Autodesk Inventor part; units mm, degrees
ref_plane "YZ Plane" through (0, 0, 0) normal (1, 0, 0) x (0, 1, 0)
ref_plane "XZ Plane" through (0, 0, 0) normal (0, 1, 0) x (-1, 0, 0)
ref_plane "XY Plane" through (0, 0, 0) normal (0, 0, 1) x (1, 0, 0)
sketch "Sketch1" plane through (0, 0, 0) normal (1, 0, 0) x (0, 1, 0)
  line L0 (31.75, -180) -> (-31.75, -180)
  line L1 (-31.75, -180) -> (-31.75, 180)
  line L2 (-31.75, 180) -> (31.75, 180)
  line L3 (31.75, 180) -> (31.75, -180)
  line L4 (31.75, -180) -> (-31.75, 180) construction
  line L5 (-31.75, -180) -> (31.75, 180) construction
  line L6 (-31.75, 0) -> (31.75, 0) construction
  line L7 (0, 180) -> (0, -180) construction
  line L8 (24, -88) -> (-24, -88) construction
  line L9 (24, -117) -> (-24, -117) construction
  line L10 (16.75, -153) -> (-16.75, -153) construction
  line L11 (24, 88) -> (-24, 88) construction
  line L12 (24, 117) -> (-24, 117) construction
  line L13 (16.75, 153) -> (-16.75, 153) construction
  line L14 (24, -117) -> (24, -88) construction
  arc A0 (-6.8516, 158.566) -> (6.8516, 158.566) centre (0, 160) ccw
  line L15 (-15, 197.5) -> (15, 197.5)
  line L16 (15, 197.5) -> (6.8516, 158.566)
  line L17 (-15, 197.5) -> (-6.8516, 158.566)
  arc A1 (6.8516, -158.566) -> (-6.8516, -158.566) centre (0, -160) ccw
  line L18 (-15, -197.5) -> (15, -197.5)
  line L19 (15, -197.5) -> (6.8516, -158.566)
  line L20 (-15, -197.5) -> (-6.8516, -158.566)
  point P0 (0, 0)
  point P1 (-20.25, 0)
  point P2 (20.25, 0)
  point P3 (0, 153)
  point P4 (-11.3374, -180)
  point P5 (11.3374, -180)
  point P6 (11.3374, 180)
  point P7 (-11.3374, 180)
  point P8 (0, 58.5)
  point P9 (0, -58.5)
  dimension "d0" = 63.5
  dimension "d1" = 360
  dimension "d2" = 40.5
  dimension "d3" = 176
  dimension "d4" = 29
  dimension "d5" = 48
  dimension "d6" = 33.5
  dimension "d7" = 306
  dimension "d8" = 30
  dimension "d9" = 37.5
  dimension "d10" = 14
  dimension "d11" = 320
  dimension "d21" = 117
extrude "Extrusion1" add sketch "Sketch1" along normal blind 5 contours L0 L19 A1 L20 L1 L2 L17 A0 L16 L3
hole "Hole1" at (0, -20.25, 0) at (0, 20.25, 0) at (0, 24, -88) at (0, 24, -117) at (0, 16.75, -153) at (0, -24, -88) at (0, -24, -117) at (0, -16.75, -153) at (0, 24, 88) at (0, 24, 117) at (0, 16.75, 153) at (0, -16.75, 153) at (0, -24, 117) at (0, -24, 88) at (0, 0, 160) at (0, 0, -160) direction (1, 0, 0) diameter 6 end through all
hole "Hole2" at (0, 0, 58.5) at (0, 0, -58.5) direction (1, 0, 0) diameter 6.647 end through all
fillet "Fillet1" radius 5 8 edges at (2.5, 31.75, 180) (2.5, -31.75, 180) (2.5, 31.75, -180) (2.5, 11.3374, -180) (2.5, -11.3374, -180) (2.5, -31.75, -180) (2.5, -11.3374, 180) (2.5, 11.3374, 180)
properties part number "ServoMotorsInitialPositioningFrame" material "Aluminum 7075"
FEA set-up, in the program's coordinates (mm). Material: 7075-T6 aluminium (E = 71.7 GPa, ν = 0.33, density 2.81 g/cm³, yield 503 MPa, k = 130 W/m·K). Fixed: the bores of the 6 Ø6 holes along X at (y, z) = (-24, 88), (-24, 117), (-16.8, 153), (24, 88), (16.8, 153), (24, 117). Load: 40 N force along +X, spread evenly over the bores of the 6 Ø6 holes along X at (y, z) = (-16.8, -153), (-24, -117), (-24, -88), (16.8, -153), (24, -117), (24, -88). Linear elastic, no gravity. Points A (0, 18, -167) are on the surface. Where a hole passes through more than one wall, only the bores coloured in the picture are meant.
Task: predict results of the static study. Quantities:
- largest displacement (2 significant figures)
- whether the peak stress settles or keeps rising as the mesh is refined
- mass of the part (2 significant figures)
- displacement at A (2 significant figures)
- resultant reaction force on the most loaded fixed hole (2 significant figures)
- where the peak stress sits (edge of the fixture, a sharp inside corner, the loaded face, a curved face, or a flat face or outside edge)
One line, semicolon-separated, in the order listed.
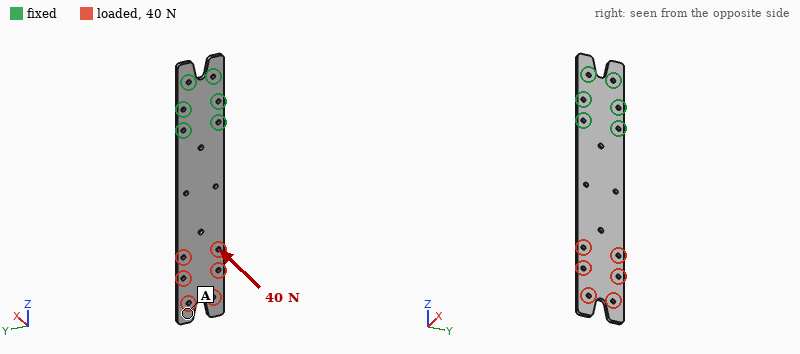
3.7 mm; keeps rising; 300 g; 3.5 mm; 66 N; edge of the fixture
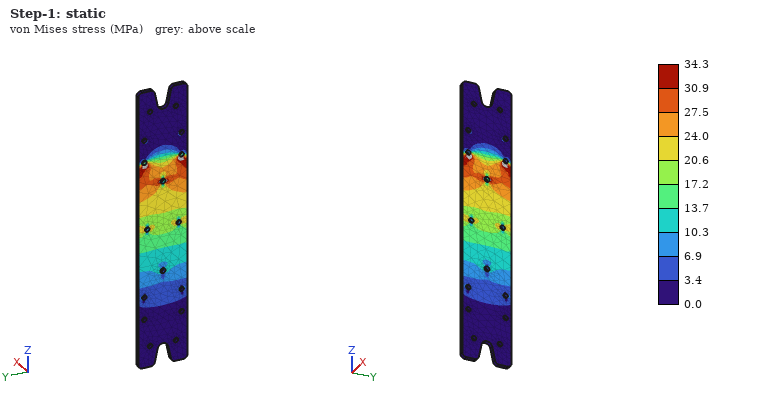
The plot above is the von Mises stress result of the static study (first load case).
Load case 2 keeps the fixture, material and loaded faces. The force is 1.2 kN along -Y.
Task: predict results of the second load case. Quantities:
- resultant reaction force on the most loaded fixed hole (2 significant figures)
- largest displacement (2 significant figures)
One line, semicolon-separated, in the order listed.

4.7 kN; 0.74 mm
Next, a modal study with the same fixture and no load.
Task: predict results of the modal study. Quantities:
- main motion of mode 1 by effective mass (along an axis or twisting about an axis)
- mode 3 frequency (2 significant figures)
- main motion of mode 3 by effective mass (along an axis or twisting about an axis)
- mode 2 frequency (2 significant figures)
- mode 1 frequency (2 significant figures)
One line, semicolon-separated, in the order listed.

along X; 470 Hz; twisting about Z; 370 Hz; 60 Hz
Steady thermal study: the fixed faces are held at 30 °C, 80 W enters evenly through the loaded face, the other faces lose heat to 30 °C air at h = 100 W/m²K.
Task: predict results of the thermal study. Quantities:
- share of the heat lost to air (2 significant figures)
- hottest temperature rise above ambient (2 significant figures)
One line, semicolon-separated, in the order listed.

97 %; 50 K
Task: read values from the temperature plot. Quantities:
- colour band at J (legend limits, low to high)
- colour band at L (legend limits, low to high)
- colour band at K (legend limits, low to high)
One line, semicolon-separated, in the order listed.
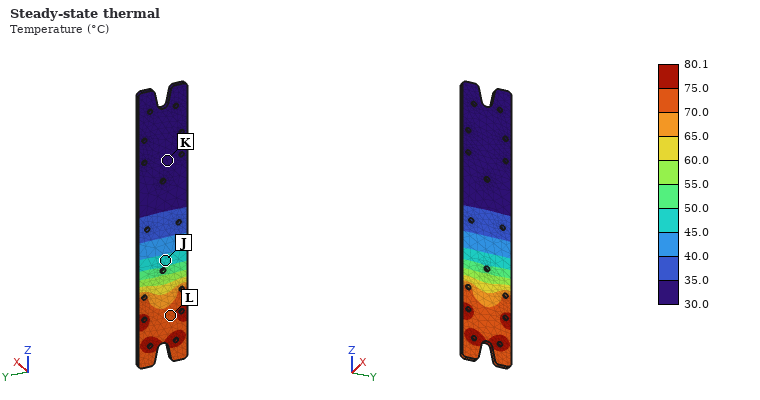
45.0 to 50.0 °C; 70.0 to 75.0 °C; 30.0 to 35.0 °C
